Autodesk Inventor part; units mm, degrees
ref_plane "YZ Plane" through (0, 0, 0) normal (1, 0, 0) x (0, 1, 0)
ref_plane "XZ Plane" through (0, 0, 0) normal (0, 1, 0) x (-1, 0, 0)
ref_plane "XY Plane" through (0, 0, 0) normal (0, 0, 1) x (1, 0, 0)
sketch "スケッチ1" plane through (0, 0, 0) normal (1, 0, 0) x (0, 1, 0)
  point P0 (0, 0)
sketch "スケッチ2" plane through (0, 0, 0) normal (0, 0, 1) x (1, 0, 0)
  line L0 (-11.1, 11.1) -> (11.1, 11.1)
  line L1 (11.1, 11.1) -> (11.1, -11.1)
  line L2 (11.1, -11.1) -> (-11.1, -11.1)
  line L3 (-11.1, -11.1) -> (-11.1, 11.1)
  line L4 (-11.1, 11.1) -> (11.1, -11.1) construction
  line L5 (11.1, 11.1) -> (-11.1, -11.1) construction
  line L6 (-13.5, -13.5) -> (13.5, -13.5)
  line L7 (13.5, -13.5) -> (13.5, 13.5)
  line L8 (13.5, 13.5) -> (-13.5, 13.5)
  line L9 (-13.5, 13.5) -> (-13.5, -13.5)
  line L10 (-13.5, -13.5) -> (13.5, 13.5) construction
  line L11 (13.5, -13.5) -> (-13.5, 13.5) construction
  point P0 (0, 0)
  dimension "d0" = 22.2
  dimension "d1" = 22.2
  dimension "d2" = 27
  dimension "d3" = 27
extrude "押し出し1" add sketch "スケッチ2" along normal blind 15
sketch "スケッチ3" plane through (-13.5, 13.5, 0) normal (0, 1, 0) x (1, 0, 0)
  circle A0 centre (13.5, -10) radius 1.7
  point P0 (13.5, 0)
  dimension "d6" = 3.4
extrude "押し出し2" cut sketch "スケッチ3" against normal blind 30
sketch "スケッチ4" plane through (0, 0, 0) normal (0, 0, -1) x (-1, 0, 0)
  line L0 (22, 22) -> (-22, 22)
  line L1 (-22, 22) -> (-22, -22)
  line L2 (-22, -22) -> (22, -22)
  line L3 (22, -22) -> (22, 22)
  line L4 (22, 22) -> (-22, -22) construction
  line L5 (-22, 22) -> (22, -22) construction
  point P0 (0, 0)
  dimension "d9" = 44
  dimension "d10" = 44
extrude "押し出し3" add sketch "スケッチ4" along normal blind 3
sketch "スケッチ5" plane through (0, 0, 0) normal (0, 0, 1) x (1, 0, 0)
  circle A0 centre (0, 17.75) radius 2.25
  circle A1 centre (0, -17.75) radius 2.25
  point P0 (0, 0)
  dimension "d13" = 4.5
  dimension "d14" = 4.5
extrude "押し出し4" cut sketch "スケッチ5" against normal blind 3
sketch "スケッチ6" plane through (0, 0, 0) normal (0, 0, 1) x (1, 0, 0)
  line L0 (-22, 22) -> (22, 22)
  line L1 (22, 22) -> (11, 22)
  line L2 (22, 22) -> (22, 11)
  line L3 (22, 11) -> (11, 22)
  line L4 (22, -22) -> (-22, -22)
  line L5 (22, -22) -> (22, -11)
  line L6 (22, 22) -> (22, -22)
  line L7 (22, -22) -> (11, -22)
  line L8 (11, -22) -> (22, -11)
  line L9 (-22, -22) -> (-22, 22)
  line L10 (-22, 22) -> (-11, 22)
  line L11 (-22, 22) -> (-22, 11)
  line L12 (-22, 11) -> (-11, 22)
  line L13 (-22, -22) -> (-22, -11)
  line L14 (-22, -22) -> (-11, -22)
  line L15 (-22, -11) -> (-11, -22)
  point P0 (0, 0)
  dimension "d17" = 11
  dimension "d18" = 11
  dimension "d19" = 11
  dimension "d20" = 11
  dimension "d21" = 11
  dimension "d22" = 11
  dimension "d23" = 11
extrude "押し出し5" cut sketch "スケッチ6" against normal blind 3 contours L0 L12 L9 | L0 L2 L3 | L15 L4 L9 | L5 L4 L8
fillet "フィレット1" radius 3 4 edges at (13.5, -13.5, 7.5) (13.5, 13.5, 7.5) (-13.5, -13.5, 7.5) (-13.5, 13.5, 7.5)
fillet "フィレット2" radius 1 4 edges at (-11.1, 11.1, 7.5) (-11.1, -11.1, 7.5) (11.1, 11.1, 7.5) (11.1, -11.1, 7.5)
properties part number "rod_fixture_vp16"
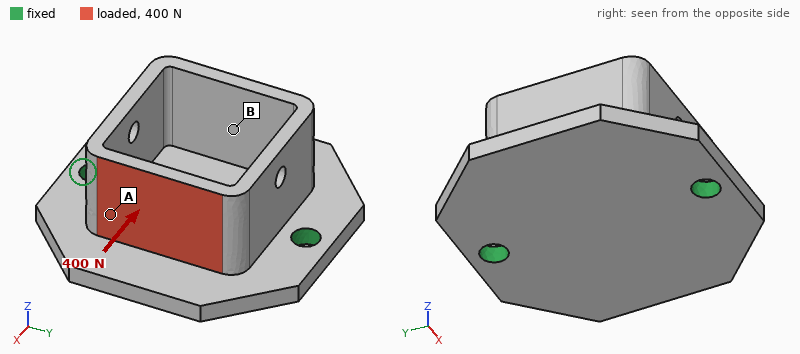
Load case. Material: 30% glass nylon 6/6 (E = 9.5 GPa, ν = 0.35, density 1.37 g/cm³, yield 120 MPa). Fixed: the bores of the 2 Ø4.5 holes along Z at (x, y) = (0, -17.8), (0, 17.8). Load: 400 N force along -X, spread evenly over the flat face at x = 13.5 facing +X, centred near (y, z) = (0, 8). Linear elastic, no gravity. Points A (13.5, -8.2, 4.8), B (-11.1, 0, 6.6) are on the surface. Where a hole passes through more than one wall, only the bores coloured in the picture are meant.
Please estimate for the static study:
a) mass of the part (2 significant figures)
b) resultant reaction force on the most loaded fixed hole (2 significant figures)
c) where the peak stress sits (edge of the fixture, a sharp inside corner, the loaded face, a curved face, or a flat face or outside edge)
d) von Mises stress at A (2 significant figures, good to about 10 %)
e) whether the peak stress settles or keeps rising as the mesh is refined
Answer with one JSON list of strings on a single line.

["11 g", "200 N", "edge of the fixture", "22 MPa", "keeps rising"]
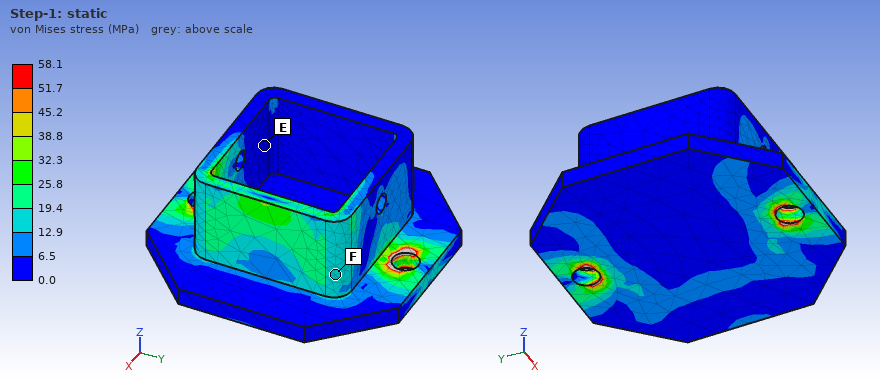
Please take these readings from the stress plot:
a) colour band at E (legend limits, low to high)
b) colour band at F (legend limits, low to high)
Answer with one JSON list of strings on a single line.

["0.0 to 6.5 MPa", "12.9 to 19.4 MPa"]
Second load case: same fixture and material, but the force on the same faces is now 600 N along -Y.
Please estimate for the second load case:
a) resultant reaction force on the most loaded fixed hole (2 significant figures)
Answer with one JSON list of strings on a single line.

["410 N"]
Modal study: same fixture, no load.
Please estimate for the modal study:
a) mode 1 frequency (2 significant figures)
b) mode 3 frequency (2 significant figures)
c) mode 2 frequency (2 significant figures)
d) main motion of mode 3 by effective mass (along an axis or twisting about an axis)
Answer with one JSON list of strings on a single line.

["2200 Hz", "5700 Hz", "5100 Hz", "along Z"]
